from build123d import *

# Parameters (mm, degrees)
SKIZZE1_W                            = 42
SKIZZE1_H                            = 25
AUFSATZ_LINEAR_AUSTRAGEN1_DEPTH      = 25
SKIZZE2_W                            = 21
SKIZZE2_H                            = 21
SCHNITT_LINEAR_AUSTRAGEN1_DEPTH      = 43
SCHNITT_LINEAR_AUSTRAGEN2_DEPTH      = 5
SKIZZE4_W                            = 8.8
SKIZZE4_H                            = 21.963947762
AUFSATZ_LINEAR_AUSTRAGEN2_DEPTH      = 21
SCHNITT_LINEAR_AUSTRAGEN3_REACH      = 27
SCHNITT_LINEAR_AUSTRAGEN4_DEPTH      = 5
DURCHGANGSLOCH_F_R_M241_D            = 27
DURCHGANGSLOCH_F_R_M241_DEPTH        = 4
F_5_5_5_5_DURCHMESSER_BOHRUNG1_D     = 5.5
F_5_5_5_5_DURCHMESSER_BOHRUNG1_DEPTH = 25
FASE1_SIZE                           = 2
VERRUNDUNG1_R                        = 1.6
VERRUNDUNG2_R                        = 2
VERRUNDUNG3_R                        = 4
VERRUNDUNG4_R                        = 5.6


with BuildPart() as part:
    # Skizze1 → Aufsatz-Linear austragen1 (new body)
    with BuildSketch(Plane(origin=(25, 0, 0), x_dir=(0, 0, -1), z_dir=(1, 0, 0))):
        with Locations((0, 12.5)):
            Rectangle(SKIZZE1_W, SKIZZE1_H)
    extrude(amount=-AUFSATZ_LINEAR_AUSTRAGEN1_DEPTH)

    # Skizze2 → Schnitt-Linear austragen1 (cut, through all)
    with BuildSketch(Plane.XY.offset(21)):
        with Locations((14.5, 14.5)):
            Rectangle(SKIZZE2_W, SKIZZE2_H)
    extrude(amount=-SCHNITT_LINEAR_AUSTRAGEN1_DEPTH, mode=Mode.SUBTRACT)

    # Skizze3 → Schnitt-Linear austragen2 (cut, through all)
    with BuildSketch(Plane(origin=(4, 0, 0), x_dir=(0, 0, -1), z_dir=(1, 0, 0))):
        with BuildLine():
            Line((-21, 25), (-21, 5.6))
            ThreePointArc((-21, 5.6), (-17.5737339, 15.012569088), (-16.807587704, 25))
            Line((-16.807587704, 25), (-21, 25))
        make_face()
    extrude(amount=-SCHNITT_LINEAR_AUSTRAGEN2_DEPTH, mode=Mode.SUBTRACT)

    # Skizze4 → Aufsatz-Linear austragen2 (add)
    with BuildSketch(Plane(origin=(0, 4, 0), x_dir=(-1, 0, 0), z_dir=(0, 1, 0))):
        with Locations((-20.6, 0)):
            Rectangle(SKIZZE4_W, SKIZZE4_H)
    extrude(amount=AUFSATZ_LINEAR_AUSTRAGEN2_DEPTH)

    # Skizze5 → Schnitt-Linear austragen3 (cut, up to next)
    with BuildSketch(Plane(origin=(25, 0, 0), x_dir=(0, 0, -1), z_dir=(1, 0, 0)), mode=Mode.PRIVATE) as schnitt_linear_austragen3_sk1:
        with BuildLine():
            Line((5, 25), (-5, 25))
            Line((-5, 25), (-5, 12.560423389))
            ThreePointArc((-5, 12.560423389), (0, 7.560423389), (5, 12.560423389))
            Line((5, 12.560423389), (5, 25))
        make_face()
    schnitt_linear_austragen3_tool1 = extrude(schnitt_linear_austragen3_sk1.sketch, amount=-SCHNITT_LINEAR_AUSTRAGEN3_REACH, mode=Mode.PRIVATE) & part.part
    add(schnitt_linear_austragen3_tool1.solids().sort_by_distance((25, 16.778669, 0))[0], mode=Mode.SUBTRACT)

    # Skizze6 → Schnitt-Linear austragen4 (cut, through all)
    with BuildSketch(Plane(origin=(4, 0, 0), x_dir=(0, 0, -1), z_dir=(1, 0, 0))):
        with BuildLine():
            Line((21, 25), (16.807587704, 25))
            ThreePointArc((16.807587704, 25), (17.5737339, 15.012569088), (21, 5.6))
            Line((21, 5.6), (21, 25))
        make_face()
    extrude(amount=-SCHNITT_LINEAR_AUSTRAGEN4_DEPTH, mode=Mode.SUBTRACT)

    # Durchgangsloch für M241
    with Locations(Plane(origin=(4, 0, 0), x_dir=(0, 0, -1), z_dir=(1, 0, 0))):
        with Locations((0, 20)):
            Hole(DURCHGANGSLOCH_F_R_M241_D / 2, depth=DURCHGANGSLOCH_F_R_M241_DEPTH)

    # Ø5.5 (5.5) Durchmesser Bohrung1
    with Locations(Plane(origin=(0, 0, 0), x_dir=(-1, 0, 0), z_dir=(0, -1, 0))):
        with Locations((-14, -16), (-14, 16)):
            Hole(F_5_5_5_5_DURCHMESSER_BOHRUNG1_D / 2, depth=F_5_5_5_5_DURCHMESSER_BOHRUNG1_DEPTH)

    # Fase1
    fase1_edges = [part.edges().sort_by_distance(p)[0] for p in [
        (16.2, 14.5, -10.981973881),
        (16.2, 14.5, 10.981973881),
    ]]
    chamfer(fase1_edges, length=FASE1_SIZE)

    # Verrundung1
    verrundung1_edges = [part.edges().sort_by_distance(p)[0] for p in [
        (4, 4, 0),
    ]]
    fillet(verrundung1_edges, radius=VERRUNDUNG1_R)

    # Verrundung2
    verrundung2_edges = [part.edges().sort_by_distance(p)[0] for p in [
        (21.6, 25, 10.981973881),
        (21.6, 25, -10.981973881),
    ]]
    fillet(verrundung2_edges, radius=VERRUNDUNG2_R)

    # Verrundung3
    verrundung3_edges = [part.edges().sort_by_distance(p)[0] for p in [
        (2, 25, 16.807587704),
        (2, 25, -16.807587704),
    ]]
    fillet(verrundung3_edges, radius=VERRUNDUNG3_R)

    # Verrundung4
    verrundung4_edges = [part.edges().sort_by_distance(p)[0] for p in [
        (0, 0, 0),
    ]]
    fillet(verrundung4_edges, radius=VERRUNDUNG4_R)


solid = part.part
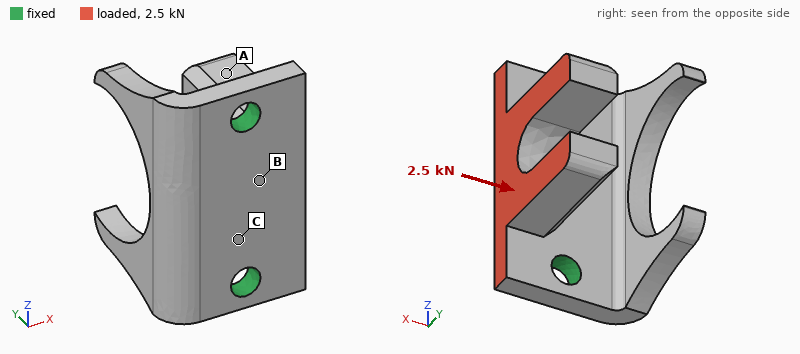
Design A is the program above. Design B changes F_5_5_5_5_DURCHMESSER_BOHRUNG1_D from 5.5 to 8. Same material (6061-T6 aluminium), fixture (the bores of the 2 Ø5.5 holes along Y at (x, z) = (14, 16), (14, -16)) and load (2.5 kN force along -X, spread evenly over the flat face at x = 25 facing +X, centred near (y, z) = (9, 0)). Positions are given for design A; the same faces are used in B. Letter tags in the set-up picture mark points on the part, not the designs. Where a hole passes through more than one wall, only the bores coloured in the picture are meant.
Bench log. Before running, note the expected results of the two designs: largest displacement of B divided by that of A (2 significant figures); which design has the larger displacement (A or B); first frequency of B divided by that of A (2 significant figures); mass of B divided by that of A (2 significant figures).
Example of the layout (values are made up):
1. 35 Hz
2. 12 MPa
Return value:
1. 0.80
2. A
3. 1.2
4. 0.97
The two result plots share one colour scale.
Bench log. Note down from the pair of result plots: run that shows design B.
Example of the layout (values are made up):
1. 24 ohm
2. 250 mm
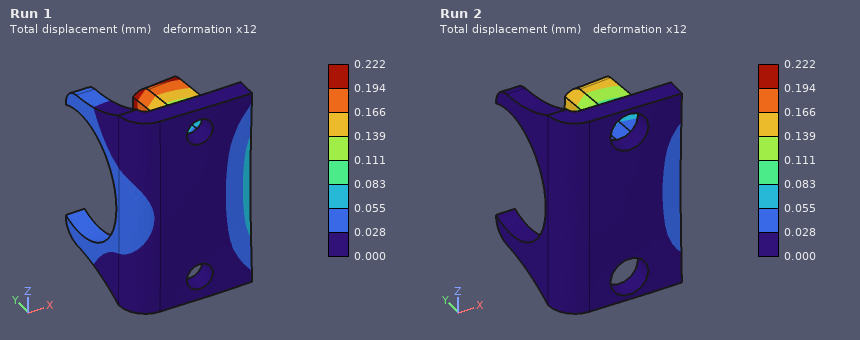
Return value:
1. Run 2
